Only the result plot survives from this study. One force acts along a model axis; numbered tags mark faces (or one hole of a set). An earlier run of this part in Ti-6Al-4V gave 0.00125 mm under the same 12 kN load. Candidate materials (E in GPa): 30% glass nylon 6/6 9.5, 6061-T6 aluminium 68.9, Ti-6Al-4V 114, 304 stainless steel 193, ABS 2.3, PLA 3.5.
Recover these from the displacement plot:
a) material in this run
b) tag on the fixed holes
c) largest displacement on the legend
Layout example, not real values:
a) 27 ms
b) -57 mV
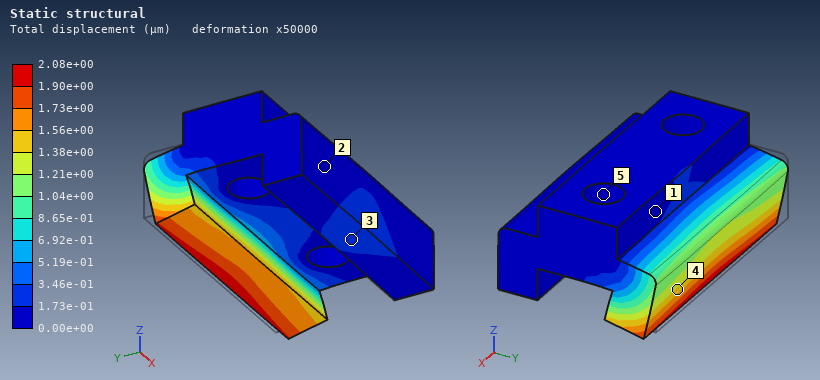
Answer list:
a) 6061-T6 aluminium
b) 5
c) 2.08e+00 µm
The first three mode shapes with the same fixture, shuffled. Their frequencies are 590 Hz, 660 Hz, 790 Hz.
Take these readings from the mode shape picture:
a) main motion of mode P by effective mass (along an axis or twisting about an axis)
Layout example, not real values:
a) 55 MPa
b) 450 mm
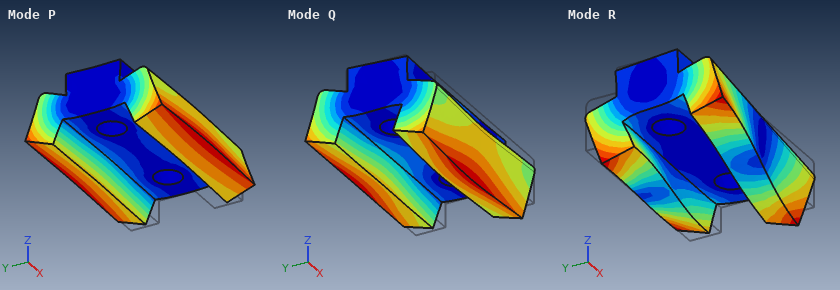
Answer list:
a) along Z
